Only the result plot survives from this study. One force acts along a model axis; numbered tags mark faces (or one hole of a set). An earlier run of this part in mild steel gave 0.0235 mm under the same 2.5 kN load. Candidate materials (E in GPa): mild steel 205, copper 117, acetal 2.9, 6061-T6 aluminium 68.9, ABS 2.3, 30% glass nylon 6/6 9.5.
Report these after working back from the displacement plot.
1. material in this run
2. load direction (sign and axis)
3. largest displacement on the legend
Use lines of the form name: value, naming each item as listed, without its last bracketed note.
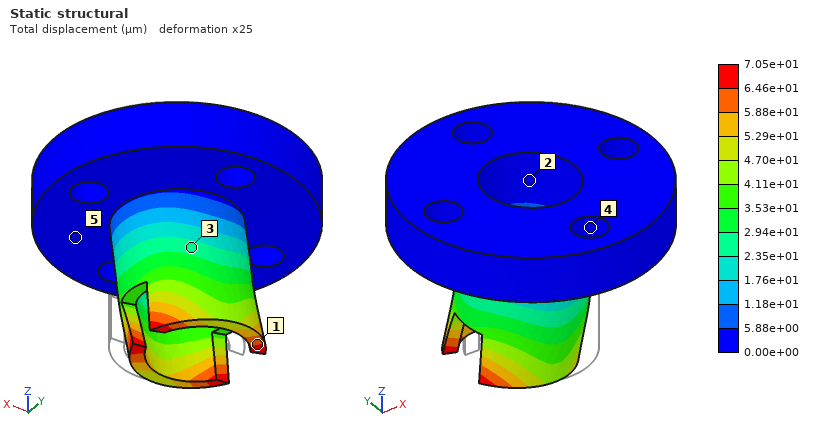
material in this run: 6061-T6 aluminium
load direction: -X
largest displacement on the legend: 7.05e+01 µm
